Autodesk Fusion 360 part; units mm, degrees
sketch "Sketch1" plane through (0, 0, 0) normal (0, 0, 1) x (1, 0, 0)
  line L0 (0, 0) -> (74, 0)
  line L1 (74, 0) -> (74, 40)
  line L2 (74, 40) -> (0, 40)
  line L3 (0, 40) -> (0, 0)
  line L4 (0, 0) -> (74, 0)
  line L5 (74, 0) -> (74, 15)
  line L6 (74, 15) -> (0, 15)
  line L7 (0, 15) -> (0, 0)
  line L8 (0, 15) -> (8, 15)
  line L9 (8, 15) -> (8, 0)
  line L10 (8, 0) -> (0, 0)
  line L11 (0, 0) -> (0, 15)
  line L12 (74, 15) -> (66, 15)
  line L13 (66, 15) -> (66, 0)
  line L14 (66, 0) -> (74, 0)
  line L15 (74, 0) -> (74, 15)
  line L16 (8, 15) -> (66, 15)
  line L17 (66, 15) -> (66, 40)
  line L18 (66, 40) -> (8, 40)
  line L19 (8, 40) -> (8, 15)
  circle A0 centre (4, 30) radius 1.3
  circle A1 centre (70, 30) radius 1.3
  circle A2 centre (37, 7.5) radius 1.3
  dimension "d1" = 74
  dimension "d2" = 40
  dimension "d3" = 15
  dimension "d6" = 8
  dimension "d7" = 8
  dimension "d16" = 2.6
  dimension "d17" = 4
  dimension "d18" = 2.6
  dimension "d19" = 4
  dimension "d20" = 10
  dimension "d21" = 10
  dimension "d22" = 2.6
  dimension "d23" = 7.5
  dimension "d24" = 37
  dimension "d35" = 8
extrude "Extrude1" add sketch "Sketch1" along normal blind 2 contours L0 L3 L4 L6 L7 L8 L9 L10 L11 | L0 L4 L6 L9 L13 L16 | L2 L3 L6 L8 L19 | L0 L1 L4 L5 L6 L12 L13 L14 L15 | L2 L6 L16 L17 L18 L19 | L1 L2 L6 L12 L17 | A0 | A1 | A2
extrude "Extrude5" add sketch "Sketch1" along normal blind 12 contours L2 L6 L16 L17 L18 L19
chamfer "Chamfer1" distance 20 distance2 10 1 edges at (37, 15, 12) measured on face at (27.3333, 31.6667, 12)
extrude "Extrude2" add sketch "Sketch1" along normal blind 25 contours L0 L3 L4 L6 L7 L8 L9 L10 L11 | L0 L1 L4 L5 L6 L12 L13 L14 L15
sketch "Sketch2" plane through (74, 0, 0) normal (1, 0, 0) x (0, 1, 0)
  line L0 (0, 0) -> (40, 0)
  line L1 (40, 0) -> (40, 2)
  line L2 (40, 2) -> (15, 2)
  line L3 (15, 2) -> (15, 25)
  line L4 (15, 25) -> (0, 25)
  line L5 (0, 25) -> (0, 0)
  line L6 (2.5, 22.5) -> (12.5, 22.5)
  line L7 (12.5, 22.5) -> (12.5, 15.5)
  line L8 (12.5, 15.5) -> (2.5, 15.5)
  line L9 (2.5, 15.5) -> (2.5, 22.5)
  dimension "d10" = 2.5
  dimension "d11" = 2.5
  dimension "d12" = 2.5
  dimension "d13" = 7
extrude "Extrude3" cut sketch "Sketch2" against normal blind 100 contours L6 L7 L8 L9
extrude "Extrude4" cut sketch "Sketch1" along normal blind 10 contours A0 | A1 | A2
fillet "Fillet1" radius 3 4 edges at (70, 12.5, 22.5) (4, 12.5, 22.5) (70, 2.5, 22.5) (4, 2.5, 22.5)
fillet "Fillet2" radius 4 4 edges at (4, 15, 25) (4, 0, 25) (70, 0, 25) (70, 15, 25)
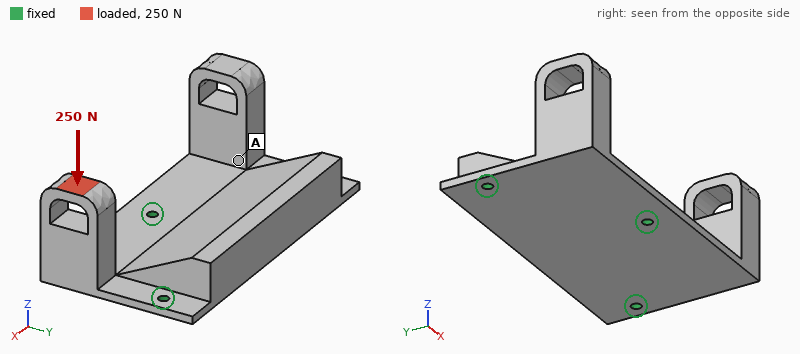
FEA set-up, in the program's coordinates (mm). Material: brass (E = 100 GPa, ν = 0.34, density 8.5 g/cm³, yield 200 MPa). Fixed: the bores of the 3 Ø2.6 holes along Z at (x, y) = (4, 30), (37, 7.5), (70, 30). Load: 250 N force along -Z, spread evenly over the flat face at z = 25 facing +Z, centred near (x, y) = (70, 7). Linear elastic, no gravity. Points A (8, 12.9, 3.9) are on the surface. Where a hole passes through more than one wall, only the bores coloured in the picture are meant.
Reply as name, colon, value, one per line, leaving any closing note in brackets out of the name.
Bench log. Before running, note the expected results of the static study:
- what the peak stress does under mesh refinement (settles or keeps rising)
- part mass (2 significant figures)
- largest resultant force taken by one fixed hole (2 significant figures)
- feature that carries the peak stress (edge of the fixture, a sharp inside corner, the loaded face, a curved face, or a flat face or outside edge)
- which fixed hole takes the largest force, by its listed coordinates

what the peak stress does under mesh refinement: keeps rising
part mass: 160 g
largest resultant force taken by one fixed hole: 340 N
feature that carries the peak stress: a sharp inside corner
which fixed hole takes the largest force, by its listed coordinates: (37, 7.5)
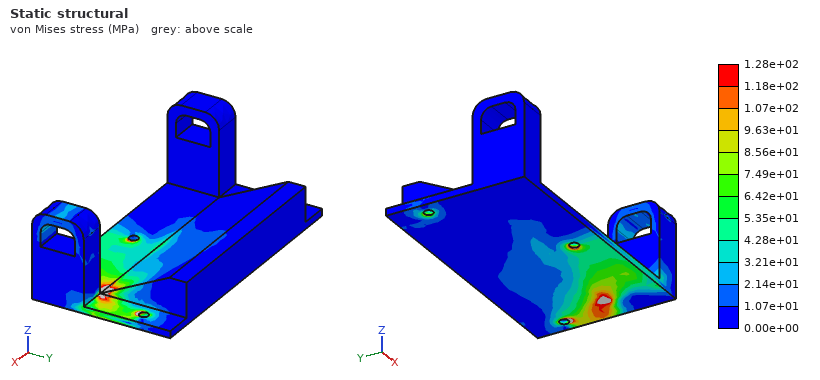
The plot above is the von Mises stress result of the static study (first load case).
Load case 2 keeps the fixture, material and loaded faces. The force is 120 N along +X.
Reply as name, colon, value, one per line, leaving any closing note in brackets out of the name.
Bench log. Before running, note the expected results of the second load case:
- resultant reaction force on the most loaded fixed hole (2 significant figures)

resultant reaction force on the most loaded fixed hole: 110 N
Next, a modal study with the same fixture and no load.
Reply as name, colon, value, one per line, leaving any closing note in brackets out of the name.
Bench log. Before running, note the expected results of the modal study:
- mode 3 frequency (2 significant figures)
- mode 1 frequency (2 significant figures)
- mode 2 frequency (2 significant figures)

mode 3 frequency: 1800 Hz
mode 1 frequency: 950 Hz
mode 2 frequency: 1000 Hz
